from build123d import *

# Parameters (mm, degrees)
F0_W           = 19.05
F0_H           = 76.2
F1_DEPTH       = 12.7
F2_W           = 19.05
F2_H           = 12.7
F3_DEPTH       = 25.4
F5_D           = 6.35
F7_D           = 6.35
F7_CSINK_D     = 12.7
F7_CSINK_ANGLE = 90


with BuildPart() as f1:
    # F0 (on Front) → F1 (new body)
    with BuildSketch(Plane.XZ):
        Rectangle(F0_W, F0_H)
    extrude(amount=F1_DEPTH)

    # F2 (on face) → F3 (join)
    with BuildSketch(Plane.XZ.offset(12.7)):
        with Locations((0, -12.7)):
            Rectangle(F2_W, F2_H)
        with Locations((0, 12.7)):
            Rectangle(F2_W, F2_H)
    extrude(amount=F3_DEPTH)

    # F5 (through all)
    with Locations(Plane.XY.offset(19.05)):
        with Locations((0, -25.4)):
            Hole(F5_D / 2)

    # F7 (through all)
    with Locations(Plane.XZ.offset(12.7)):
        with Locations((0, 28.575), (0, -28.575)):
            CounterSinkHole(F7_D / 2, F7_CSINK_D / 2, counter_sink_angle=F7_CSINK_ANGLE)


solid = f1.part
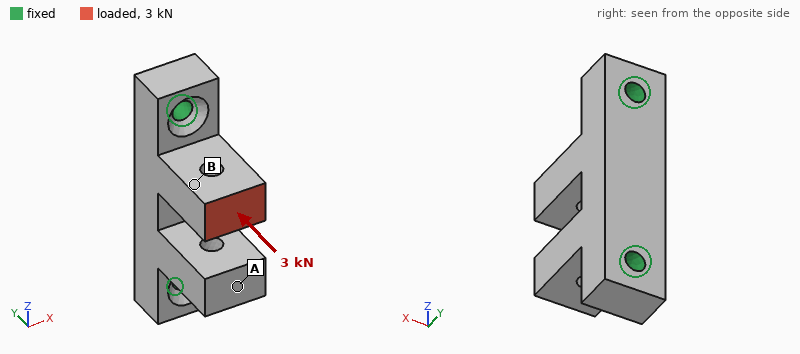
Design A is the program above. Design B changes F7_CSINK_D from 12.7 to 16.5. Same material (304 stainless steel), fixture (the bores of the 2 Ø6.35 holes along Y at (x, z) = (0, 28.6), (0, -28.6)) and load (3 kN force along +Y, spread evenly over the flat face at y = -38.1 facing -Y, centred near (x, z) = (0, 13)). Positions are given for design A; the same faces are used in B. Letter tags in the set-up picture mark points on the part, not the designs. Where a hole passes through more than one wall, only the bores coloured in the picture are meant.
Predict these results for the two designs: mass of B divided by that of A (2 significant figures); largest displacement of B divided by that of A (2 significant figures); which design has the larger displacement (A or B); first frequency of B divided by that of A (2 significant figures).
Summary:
0.98
1.1
B
0.88
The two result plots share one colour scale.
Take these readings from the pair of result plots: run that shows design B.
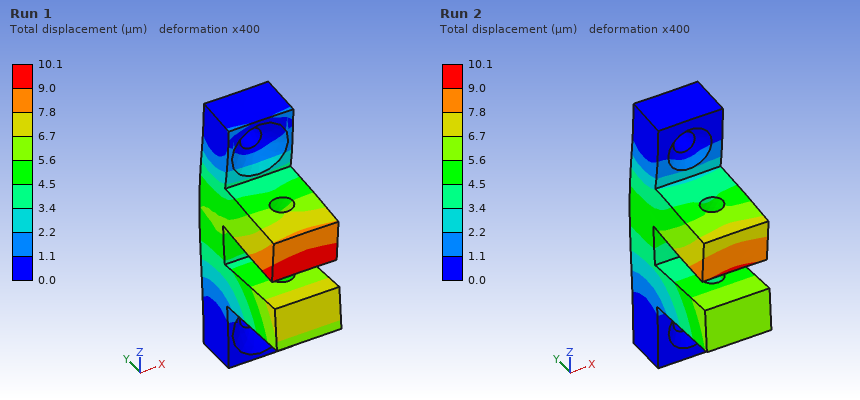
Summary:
Run 1
